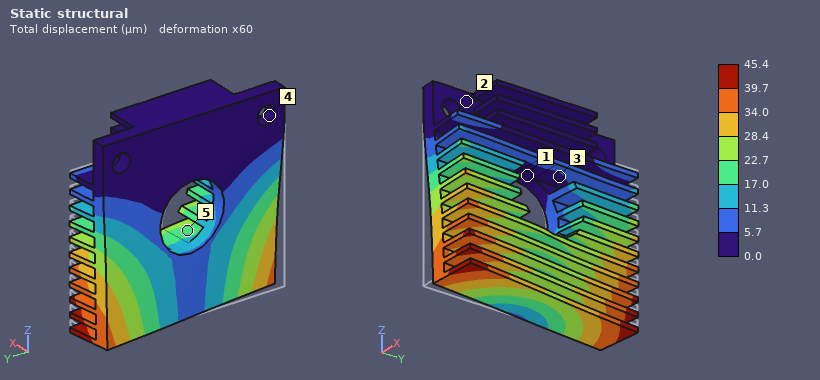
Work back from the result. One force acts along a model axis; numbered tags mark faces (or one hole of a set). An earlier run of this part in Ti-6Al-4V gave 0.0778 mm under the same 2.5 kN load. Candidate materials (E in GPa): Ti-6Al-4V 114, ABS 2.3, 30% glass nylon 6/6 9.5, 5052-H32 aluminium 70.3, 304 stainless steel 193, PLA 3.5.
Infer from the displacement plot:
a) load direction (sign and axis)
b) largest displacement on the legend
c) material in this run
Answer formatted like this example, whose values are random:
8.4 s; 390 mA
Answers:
+Y; 45.4 µm; 304 stainless steel
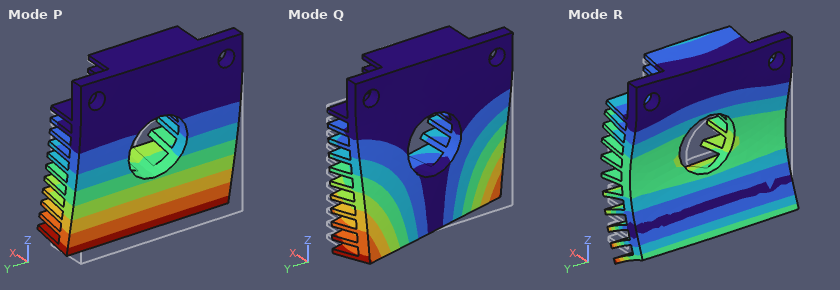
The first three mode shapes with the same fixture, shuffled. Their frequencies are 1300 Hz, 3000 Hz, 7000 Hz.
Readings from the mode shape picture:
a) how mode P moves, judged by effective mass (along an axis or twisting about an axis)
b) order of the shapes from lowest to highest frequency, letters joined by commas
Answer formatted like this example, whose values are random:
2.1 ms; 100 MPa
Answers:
along X; P, Q, R
